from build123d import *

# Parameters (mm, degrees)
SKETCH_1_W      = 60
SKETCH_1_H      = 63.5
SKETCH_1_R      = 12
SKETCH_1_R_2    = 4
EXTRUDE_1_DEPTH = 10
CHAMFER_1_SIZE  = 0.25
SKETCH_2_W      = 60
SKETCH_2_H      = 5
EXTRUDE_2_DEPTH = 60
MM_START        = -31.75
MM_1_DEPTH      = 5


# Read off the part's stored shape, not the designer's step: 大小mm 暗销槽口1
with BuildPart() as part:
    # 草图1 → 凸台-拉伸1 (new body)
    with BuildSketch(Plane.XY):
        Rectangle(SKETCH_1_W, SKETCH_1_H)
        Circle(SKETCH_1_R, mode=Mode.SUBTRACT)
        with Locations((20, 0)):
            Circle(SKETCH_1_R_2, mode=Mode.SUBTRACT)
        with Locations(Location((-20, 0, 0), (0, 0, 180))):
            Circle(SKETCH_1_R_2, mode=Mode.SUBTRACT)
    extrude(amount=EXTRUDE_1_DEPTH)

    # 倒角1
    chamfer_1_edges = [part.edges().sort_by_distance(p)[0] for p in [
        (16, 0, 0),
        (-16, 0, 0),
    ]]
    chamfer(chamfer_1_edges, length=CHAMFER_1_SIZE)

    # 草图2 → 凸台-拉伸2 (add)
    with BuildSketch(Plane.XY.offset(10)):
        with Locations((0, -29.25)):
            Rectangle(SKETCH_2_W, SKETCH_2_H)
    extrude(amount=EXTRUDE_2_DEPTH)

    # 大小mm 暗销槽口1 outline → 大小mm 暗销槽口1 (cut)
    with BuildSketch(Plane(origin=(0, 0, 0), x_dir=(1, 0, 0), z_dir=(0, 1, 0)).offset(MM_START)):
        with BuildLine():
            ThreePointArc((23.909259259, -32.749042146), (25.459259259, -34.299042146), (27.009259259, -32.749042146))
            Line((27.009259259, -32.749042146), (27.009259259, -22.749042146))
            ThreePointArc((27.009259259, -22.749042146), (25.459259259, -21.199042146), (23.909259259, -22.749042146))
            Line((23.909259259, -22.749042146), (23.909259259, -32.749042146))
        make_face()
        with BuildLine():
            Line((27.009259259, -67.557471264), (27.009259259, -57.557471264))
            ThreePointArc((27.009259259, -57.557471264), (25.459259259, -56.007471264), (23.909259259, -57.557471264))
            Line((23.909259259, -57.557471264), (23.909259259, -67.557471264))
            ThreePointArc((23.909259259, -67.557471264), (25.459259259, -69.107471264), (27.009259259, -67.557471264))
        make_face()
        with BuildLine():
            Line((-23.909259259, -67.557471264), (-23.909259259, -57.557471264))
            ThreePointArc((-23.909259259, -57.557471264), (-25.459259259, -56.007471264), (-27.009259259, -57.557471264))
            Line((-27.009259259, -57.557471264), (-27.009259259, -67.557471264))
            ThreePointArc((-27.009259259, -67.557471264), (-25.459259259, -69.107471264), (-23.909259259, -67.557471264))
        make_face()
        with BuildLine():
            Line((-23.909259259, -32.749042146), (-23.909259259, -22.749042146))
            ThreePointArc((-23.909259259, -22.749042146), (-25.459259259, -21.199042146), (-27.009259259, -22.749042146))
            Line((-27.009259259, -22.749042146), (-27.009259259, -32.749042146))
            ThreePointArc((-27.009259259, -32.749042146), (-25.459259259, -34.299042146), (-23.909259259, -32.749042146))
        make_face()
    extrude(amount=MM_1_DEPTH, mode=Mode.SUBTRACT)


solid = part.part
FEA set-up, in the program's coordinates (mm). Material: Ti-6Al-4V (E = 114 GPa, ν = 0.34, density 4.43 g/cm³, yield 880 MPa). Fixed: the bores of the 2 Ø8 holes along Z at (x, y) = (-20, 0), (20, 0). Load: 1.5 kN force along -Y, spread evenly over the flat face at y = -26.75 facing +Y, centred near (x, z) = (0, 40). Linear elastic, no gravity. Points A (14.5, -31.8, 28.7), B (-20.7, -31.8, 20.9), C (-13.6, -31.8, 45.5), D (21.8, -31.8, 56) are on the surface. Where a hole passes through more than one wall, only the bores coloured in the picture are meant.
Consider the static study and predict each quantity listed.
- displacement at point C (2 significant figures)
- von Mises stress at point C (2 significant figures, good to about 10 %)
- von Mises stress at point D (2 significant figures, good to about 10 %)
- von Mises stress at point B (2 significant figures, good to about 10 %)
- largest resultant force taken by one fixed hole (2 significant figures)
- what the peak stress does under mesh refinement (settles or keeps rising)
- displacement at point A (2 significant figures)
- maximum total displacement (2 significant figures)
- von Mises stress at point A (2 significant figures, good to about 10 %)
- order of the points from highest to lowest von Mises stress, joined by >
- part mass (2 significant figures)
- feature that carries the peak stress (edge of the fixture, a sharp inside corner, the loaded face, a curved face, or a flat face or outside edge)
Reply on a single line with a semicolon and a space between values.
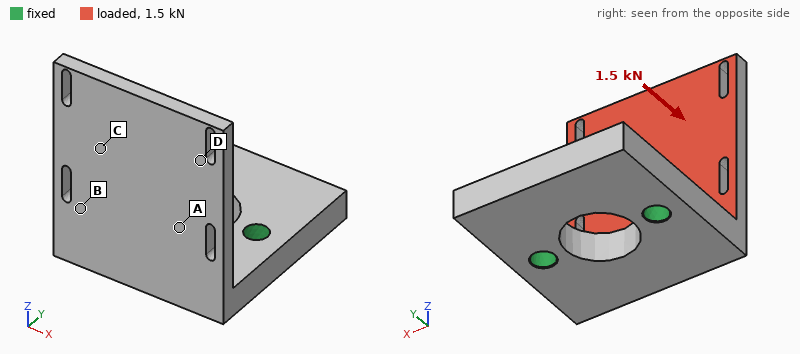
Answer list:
0.44 mm; 29 MPa; 15 MPa; 120 MPa; 840 N; keeps rising; 0.20 mm; 0.84 mm; 85 MPa; B > A > C > D; 220 g; edge of the fixture
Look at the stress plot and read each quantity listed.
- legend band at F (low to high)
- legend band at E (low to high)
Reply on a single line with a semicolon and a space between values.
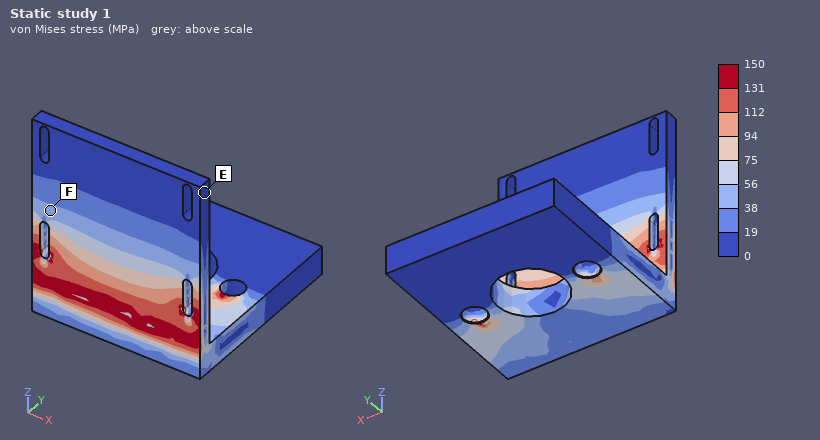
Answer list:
38 to 56 MPa; 0 to 19 MPa
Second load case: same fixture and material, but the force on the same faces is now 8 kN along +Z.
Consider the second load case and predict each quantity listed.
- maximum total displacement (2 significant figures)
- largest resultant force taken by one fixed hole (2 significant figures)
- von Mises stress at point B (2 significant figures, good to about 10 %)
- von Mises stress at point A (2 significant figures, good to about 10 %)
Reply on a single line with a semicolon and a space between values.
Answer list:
0.18 mm; 4.0 kN; 41 MPa; 37 MPa
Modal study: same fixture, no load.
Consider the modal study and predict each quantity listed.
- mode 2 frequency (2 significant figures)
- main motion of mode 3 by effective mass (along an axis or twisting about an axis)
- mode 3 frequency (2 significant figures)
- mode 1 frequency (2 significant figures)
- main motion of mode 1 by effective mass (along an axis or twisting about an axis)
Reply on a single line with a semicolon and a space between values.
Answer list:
2400 Hz; along X; 3000 Hz; 960 Hz; along Y
